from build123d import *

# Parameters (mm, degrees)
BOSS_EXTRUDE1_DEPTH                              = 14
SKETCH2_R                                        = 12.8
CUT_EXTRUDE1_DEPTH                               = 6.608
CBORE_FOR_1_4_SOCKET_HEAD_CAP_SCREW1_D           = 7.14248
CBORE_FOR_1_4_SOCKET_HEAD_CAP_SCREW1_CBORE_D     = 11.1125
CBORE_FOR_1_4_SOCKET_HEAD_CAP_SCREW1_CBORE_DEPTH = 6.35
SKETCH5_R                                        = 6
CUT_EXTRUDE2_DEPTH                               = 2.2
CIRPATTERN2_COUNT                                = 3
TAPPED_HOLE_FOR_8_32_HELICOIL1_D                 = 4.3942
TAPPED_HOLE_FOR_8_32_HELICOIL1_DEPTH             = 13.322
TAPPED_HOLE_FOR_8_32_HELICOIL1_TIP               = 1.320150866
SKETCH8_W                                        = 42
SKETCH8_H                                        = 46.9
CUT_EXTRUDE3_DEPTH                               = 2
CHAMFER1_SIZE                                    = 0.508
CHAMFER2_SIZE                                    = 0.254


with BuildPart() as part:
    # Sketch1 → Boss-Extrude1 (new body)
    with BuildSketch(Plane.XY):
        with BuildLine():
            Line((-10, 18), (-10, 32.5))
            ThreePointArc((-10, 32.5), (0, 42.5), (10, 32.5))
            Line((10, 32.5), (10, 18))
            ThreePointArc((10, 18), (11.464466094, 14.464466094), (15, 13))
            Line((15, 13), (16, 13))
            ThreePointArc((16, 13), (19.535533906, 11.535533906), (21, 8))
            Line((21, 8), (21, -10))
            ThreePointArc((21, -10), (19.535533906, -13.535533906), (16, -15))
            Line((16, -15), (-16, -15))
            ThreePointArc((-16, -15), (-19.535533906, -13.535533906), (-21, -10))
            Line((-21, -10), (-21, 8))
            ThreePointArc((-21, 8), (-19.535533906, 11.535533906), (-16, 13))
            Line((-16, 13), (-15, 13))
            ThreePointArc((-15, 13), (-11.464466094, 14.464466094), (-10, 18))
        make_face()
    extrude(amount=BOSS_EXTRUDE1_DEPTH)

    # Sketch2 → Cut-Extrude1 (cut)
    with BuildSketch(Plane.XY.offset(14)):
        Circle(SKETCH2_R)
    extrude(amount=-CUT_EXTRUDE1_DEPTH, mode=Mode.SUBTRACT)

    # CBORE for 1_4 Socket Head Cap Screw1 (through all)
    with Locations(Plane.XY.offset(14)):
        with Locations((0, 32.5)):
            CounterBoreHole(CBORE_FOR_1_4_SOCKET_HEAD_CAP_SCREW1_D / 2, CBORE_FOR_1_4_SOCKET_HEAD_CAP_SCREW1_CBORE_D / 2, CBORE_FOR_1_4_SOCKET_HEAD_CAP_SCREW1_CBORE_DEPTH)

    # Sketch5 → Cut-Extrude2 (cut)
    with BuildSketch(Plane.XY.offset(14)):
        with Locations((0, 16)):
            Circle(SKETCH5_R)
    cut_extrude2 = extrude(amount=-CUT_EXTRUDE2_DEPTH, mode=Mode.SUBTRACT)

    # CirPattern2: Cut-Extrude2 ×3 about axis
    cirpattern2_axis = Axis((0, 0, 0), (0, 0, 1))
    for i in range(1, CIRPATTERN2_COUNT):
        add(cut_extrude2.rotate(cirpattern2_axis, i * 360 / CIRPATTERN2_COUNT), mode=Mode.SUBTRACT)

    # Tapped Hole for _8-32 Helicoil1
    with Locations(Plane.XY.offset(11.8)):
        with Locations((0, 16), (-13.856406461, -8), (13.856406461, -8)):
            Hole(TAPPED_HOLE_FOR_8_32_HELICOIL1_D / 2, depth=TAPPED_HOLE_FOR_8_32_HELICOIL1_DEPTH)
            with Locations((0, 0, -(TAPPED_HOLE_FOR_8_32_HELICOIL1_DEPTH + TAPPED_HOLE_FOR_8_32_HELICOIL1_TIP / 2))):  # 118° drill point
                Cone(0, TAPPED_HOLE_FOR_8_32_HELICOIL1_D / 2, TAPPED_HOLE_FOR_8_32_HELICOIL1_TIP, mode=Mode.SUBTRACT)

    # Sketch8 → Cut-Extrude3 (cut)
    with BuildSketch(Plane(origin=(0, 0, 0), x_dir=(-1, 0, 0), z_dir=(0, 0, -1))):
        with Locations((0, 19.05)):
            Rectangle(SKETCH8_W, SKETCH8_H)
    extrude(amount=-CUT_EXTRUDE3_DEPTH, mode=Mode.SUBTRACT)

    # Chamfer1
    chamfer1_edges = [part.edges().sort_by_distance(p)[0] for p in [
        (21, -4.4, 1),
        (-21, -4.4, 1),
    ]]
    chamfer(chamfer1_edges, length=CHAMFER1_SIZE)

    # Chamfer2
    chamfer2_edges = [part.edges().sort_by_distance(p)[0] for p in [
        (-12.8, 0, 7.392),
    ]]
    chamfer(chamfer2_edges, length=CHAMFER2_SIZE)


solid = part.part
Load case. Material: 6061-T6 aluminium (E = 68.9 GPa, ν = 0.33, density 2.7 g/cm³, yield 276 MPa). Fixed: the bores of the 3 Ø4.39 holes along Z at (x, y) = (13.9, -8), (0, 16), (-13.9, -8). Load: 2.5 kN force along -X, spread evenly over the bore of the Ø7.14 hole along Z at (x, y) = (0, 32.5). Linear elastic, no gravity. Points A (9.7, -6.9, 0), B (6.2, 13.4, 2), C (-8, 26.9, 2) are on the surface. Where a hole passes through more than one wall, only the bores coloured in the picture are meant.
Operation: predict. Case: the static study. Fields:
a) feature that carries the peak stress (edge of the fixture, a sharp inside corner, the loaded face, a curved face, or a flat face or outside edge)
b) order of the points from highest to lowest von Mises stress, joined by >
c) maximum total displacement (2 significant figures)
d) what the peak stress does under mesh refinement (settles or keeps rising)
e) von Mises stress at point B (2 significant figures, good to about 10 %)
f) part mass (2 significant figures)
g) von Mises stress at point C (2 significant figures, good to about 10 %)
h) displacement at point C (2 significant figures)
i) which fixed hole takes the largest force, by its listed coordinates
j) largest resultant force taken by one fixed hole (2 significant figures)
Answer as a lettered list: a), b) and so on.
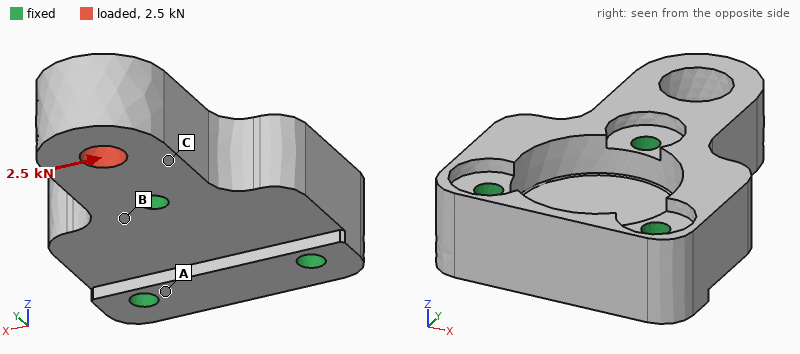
a) edge of the fixture
b) C > B > A
c) 47 µm
d) keeps rising
e) 20 MPa
f) 43 g
g) 33 MPa
h) 21 µm
i) (0, 16)
j) 2.6 kN
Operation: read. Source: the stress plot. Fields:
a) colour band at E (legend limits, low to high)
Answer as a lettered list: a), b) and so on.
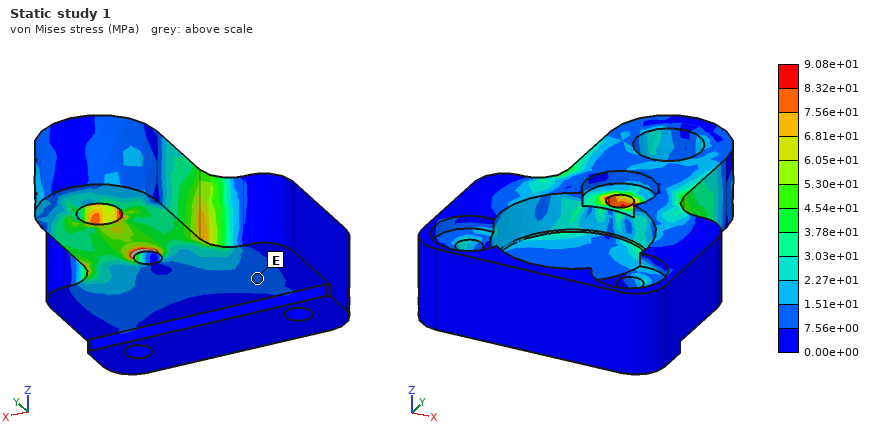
a) 7.56e+00 to 1.51e+01 MPa
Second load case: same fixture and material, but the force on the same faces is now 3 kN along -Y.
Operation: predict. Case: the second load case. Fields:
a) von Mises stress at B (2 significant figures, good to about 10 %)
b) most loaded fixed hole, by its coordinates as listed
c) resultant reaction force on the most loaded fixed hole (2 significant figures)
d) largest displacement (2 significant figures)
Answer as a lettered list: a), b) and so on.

a) 12 MPa
b) (0, 16)
c) 2.4 kN
d) 21 µm
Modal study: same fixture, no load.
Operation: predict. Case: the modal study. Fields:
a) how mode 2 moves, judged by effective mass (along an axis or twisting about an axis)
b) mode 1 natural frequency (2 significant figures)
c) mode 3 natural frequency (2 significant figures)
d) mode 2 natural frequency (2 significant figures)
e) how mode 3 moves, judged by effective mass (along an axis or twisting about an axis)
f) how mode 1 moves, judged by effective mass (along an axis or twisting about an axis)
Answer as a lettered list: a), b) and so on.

a) along X
b) 12 kHz
c) 21 kHz
d) 15 kHz
e) twisting about Y
f) along Z
